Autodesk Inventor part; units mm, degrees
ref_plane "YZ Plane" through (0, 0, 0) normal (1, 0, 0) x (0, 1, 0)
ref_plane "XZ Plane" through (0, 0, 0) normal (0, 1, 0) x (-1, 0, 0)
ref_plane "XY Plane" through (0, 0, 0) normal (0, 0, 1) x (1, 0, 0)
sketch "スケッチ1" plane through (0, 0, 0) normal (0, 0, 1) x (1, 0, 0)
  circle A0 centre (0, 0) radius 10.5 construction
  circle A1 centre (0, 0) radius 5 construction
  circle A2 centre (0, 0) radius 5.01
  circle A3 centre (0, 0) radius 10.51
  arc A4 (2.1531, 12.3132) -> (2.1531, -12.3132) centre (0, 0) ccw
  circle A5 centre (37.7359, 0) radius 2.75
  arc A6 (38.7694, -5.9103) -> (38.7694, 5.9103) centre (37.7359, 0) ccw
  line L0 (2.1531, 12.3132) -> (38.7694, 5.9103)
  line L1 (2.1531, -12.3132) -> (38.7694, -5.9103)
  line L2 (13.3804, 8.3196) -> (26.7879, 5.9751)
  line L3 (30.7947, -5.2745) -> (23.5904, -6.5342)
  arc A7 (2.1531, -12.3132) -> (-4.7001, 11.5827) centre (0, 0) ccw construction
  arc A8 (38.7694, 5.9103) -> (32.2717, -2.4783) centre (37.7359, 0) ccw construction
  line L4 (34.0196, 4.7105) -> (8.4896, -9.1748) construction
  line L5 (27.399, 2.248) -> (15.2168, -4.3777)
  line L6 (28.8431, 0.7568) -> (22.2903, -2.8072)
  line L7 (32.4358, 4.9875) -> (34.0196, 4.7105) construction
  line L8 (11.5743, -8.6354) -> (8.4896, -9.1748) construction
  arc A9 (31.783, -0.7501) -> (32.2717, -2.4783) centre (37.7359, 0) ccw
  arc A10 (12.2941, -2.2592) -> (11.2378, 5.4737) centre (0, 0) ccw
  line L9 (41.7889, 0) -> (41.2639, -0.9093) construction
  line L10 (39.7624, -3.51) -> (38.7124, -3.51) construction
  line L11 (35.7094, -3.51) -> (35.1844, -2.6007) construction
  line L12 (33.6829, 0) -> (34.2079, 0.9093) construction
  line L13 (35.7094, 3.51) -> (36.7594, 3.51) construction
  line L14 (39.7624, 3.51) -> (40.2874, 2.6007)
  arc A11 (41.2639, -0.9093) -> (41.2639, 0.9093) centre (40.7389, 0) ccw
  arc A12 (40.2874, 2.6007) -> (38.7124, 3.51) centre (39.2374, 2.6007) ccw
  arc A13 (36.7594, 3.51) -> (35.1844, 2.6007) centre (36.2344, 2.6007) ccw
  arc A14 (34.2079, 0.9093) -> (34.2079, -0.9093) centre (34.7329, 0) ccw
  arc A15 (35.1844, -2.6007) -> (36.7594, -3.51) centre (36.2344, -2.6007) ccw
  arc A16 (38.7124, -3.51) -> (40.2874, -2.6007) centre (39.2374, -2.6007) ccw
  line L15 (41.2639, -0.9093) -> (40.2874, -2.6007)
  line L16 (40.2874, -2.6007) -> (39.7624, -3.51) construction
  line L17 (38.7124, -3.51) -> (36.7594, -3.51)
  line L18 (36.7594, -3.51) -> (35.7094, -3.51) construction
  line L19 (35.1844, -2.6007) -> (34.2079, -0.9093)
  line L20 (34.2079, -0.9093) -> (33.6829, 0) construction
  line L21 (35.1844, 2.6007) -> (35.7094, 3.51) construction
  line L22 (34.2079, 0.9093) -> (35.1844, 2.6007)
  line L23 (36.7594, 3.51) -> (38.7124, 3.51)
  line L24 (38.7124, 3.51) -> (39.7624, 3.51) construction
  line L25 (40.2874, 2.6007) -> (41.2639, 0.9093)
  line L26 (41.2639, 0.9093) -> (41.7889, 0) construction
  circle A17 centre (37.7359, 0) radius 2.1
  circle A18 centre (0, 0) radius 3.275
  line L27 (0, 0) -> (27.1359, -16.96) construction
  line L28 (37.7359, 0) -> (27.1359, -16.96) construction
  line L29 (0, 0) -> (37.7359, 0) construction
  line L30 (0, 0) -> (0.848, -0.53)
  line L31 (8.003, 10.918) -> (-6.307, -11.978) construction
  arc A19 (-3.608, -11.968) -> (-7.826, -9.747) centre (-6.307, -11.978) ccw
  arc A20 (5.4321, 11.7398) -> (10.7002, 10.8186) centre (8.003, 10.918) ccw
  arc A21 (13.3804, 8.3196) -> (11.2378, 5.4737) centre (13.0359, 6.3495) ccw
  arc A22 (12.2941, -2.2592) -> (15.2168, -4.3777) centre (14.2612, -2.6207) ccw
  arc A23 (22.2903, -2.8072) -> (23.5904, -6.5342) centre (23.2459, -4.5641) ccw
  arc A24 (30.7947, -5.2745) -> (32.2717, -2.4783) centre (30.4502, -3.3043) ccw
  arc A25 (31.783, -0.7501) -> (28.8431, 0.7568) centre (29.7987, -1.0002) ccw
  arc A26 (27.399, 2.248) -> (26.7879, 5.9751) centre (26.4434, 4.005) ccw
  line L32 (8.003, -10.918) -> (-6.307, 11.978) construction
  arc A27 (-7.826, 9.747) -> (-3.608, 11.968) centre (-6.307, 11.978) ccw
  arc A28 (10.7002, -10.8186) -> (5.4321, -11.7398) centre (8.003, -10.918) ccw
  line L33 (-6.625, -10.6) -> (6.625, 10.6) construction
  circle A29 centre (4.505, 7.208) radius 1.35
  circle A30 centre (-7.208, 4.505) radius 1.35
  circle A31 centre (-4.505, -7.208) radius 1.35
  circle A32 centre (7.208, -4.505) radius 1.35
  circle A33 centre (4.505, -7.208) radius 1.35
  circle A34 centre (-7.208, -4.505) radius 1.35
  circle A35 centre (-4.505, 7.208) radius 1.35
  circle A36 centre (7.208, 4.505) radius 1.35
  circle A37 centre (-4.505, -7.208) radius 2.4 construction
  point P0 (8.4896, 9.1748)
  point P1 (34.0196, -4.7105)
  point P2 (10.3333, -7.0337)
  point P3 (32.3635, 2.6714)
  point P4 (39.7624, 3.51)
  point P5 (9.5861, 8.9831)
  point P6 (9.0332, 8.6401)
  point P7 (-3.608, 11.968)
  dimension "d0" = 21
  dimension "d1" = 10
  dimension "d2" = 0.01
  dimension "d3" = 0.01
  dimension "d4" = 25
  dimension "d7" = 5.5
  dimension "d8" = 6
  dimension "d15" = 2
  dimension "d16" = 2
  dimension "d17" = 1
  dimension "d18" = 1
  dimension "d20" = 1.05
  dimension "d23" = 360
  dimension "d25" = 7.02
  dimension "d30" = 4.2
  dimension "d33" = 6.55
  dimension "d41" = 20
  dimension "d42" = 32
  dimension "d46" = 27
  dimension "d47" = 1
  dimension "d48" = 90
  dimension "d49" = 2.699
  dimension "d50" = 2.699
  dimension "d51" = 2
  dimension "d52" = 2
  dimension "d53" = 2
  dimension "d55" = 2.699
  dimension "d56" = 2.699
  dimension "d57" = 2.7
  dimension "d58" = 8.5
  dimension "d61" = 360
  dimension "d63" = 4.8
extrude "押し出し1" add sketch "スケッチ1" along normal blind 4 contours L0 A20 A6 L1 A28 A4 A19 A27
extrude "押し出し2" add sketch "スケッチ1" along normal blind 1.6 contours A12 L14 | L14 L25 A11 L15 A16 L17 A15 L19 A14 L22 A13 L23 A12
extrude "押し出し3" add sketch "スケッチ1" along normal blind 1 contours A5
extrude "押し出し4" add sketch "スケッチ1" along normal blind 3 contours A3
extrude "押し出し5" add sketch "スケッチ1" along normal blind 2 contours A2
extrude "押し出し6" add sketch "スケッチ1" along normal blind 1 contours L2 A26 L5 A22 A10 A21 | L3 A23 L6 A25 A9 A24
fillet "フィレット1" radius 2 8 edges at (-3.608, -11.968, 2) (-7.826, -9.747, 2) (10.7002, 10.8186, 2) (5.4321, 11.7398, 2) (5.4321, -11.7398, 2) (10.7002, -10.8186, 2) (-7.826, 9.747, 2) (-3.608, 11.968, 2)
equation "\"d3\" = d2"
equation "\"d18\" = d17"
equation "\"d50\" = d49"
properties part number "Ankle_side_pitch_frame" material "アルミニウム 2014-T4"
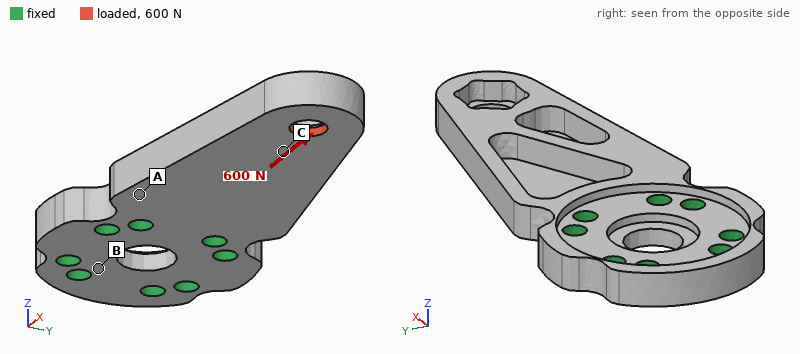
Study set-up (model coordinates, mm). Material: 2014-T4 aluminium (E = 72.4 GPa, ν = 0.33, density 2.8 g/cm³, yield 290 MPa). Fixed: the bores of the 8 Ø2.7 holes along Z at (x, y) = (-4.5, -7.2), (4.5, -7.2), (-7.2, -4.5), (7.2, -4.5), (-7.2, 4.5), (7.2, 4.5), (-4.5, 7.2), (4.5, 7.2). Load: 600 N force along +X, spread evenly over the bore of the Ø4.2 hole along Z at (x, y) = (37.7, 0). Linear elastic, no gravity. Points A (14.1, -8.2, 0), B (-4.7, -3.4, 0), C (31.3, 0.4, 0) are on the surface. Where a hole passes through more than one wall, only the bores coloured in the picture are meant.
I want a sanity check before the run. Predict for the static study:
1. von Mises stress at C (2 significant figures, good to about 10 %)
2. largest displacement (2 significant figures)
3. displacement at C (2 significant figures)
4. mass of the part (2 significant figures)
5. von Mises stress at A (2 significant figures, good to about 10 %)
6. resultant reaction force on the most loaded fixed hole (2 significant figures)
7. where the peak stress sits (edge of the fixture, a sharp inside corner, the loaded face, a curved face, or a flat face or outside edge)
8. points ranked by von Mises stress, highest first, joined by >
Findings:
40 MPa
0.10 mm
0.045 mm
7.1 g
23 MPa
240 N
a sharp inside corner
C > A > B
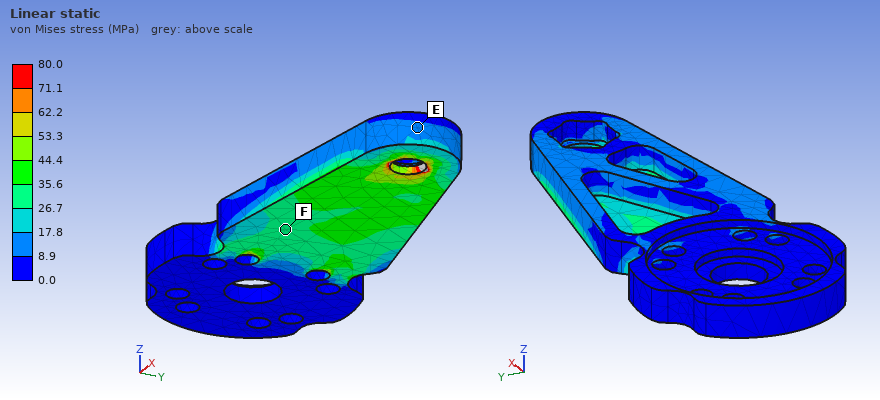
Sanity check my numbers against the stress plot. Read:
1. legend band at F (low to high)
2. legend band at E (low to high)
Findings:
26.7 to 35.6 MPa
8.9 to 17.8 MPa
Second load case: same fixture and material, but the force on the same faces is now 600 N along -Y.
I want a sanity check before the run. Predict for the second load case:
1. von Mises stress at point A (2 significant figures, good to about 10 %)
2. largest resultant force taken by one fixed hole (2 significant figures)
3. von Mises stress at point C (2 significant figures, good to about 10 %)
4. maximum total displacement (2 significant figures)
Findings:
70 MPa
870 N
62 MPa
0.14 mm
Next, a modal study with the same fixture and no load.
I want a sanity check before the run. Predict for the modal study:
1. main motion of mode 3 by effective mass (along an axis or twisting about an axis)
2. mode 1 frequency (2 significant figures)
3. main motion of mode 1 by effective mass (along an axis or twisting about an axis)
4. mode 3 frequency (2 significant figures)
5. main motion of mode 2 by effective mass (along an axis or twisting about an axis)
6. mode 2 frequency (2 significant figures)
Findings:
along Y
2600 Hz
along Z
11 kHz
along Y
9200 Hz
